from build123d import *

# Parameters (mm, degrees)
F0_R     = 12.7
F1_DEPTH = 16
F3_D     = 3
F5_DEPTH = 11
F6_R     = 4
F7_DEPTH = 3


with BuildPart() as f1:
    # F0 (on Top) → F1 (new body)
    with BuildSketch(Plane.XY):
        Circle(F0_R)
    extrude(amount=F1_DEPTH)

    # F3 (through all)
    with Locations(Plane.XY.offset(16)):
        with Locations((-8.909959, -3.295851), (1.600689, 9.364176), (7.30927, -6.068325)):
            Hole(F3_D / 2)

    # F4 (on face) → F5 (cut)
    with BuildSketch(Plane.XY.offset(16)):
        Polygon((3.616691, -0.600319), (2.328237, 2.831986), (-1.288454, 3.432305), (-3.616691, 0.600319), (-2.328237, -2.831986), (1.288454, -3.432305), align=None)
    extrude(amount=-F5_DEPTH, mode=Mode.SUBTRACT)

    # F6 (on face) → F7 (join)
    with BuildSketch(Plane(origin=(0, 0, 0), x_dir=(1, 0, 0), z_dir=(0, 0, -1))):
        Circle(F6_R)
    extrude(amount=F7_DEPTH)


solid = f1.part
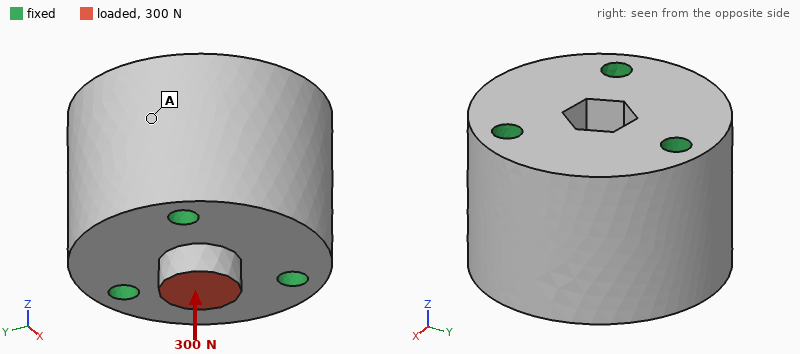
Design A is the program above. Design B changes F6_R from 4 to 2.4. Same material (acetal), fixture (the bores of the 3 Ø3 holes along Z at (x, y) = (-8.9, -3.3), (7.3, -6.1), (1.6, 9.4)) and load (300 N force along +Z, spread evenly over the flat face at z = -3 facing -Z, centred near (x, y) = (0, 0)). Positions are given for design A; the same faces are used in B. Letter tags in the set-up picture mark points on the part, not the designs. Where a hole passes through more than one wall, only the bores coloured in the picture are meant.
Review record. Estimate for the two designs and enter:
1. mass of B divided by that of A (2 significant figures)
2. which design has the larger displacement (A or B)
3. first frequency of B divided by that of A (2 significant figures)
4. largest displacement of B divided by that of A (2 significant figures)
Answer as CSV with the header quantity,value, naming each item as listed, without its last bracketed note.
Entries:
quantity,value
mass of B divided by that of A,0.99
which design has the larger displacement,B
first frequency of B divided by that of A,1.0
largest displacement of B divided by that of A,2.2
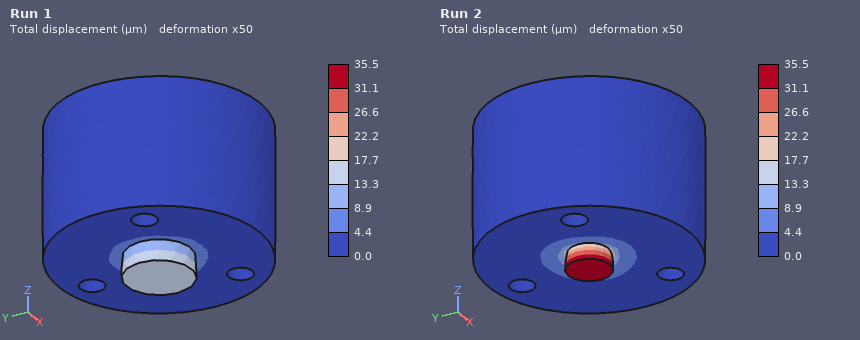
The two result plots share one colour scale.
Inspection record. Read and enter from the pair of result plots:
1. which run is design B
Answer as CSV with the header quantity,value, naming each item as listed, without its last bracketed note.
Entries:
quantity,value
which run is design B,Run 2
